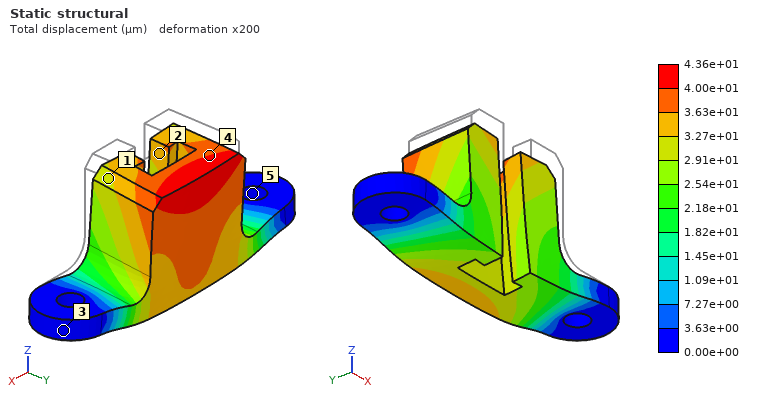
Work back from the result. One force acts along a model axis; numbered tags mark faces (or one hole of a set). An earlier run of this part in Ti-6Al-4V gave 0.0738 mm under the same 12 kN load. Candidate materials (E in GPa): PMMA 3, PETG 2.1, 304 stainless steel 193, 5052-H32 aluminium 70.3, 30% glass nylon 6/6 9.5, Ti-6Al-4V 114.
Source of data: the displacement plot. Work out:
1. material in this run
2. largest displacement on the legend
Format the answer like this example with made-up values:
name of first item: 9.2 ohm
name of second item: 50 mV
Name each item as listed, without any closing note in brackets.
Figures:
material in this run: 304 stainless steel
largest displacement on the legend: 4.36e+01 µm
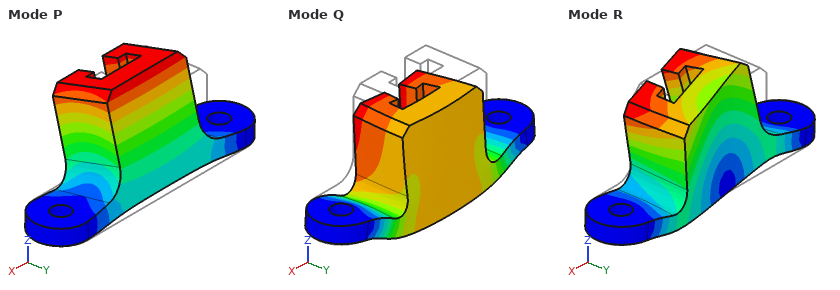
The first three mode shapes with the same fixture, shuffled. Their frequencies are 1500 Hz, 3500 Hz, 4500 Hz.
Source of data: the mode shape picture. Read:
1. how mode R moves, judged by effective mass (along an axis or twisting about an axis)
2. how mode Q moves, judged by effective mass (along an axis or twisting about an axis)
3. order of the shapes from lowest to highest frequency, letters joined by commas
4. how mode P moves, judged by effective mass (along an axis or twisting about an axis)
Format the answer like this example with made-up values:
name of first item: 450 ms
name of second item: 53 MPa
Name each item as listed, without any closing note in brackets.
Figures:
how mode R moves, judged by effective mass: along X
how mode Q moves, judged by effective mass: along Z
order of the shapes from lowest to highest frequency, letters joined by commas: P, Q, R
how mode P moves, judged by effective mass: along Y
